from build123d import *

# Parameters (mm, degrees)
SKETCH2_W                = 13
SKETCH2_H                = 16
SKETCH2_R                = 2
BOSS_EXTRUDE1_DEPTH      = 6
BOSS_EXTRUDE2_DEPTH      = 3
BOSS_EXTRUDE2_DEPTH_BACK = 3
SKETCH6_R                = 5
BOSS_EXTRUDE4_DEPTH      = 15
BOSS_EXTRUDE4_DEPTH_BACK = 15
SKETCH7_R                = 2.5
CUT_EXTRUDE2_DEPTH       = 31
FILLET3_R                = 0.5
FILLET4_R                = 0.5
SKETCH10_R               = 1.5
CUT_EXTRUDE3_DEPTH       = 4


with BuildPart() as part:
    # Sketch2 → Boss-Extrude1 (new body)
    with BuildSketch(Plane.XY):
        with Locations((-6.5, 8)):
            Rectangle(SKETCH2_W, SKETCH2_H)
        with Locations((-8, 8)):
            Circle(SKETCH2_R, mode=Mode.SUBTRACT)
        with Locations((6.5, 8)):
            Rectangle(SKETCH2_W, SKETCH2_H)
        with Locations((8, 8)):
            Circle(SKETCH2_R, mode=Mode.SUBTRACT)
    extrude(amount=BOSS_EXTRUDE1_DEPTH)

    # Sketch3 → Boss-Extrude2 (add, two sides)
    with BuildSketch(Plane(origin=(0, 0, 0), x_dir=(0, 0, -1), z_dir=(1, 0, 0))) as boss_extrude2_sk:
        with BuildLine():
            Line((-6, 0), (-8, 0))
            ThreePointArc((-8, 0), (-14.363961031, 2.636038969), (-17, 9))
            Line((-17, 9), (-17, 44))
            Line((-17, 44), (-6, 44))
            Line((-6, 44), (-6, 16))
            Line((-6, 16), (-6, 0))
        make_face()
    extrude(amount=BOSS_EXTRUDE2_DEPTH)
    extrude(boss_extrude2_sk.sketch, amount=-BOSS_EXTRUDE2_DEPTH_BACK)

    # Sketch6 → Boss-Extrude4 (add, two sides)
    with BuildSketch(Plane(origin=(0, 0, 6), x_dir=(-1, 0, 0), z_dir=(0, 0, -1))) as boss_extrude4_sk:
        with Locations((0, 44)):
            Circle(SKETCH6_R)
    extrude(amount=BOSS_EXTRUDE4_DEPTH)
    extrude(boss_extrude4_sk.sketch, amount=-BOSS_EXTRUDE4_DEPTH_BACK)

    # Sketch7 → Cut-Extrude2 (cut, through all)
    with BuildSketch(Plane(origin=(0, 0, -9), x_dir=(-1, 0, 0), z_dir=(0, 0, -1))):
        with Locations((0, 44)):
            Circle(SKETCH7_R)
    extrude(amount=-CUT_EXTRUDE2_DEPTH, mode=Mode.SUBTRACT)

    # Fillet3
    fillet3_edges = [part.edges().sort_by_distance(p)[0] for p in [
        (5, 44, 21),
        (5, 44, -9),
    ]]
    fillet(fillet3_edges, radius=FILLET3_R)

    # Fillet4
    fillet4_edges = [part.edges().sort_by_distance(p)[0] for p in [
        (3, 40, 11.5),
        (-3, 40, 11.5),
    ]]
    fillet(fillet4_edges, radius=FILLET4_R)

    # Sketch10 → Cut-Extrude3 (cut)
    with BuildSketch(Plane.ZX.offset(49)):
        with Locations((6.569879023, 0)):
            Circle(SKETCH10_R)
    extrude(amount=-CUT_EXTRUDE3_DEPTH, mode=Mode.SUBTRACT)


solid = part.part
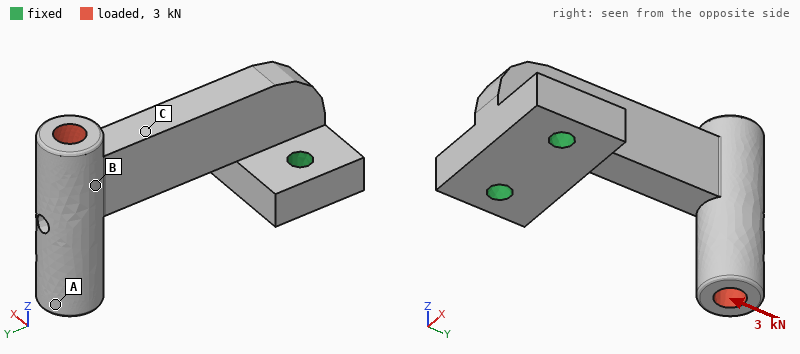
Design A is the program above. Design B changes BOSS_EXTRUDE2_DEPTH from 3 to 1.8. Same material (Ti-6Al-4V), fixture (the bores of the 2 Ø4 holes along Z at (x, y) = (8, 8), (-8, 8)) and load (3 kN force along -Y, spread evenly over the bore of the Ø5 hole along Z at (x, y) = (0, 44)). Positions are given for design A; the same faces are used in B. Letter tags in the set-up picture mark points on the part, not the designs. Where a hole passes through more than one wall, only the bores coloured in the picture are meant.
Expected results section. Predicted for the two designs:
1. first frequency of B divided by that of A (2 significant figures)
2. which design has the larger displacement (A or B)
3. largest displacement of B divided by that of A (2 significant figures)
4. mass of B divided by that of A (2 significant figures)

0.75
B
1.3
0.92
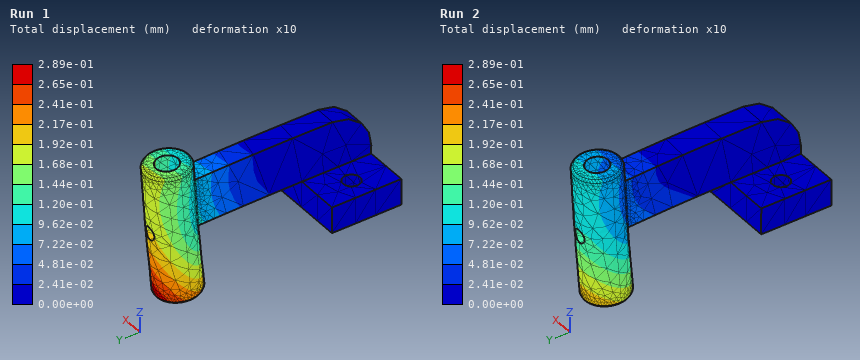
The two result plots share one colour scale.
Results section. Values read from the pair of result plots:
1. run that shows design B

Run 1
